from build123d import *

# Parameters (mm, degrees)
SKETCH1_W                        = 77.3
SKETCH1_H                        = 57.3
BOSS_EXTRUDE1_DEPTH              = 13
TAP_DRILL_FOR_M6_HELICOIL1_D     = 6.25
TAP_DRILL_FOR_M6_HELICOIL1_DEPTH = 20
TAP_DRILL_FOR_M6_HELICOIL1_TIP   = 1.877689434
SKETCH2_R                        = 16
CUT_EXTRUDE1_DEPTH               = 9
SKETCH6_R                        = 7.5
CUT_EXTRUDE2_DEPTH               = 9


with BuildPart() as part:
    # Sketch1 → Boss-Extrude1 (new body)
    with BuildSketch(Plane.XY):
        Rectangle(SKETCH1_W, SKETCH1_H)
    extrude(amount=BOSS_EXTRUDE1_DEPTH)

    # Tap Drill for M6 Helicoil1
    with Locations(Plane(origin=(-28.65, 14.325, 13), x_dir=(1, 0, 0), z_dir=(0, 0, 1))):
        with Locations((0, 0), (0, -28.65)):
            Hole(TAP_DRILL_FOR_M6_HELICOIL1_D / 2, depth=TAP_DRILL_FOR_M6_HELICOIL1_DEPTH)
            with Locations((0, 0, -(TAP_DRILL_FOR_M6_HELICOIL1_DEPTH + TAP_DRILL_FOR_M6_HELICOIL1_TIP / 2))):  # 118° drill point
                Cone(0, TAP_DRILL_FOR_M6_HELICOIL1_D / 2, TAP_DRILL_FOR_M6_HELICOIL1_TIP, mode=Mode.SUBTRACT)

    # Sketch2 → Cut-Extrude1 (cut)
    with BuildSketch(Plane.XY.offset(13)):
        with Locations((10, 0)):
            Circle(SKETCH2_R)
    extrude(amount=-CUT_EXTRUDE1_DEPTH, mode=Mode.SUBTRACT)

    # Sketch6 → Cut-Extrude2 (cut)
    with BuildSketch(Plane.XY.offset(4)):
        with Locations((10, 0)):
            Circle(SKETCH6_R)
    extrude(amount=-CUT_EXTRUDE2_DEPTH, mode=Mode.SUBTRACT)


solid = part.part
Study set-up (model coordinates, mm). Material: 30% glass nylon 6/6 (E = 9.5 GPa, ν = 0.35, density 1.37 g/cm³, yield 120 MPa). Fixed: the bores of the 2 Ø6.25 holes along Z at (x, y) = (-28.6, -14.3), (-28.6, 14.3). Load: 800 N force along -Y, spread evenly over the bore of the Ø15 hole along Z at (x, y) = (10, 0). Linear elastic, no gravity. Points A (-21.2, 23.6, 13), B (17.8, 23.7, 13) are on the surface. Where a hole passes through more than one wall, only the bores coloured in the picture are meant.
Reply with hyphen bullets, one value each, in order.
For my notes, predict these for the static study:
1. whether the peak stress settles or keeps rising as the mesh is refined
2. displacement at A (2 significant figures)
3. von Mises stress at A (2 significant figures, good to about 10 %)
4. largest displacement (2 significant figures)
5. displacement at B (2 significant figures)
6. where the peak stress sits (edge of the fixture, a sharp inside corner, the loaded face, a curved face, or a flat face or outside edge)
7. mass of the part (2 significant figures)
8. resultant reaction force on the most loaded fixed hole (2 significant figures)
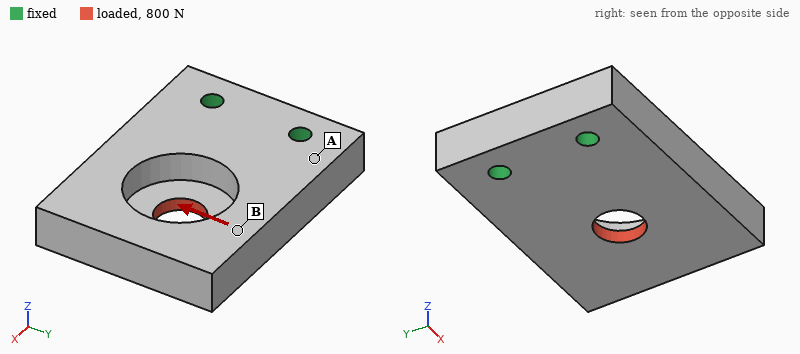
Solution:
- keeps rising
- 11 µm
- 2.8 MPa
- 68 µm
- 45 µm
- edge of the fixture
- 67 g
- 990 N
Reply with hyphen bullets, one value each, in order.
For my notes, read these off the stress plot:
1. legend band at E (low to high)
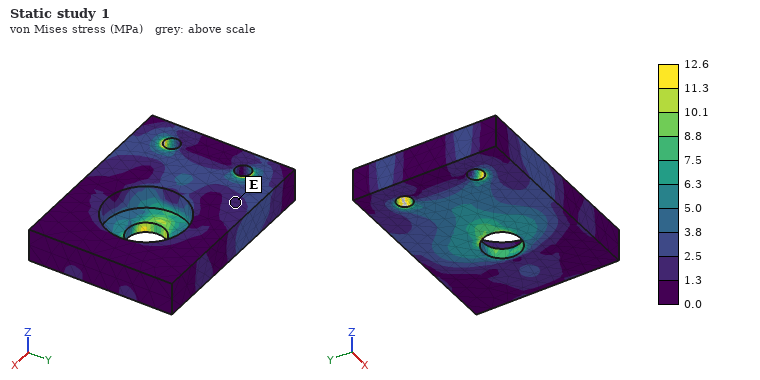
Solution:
- 1.3 to 2.5 MPa
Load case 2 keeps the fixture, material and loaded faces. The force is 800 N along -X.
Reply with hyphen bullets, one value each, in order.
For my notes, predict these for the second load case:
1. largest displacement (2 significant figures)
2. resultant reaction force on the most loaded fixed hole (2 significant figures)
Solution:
- 70 µm
- 400 N
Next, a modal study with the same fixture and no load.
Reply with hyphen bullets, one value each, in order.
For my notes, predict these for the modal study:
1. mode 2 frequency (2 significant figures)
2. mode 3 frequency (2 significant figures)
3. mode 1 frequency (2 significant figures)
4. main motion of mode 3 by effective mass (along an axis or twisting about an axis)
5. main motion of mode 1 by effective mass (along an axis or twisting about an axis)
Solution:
- 2400 Hz
- 3000 Hz
- 1100 Hz
- along Y
- along Z
